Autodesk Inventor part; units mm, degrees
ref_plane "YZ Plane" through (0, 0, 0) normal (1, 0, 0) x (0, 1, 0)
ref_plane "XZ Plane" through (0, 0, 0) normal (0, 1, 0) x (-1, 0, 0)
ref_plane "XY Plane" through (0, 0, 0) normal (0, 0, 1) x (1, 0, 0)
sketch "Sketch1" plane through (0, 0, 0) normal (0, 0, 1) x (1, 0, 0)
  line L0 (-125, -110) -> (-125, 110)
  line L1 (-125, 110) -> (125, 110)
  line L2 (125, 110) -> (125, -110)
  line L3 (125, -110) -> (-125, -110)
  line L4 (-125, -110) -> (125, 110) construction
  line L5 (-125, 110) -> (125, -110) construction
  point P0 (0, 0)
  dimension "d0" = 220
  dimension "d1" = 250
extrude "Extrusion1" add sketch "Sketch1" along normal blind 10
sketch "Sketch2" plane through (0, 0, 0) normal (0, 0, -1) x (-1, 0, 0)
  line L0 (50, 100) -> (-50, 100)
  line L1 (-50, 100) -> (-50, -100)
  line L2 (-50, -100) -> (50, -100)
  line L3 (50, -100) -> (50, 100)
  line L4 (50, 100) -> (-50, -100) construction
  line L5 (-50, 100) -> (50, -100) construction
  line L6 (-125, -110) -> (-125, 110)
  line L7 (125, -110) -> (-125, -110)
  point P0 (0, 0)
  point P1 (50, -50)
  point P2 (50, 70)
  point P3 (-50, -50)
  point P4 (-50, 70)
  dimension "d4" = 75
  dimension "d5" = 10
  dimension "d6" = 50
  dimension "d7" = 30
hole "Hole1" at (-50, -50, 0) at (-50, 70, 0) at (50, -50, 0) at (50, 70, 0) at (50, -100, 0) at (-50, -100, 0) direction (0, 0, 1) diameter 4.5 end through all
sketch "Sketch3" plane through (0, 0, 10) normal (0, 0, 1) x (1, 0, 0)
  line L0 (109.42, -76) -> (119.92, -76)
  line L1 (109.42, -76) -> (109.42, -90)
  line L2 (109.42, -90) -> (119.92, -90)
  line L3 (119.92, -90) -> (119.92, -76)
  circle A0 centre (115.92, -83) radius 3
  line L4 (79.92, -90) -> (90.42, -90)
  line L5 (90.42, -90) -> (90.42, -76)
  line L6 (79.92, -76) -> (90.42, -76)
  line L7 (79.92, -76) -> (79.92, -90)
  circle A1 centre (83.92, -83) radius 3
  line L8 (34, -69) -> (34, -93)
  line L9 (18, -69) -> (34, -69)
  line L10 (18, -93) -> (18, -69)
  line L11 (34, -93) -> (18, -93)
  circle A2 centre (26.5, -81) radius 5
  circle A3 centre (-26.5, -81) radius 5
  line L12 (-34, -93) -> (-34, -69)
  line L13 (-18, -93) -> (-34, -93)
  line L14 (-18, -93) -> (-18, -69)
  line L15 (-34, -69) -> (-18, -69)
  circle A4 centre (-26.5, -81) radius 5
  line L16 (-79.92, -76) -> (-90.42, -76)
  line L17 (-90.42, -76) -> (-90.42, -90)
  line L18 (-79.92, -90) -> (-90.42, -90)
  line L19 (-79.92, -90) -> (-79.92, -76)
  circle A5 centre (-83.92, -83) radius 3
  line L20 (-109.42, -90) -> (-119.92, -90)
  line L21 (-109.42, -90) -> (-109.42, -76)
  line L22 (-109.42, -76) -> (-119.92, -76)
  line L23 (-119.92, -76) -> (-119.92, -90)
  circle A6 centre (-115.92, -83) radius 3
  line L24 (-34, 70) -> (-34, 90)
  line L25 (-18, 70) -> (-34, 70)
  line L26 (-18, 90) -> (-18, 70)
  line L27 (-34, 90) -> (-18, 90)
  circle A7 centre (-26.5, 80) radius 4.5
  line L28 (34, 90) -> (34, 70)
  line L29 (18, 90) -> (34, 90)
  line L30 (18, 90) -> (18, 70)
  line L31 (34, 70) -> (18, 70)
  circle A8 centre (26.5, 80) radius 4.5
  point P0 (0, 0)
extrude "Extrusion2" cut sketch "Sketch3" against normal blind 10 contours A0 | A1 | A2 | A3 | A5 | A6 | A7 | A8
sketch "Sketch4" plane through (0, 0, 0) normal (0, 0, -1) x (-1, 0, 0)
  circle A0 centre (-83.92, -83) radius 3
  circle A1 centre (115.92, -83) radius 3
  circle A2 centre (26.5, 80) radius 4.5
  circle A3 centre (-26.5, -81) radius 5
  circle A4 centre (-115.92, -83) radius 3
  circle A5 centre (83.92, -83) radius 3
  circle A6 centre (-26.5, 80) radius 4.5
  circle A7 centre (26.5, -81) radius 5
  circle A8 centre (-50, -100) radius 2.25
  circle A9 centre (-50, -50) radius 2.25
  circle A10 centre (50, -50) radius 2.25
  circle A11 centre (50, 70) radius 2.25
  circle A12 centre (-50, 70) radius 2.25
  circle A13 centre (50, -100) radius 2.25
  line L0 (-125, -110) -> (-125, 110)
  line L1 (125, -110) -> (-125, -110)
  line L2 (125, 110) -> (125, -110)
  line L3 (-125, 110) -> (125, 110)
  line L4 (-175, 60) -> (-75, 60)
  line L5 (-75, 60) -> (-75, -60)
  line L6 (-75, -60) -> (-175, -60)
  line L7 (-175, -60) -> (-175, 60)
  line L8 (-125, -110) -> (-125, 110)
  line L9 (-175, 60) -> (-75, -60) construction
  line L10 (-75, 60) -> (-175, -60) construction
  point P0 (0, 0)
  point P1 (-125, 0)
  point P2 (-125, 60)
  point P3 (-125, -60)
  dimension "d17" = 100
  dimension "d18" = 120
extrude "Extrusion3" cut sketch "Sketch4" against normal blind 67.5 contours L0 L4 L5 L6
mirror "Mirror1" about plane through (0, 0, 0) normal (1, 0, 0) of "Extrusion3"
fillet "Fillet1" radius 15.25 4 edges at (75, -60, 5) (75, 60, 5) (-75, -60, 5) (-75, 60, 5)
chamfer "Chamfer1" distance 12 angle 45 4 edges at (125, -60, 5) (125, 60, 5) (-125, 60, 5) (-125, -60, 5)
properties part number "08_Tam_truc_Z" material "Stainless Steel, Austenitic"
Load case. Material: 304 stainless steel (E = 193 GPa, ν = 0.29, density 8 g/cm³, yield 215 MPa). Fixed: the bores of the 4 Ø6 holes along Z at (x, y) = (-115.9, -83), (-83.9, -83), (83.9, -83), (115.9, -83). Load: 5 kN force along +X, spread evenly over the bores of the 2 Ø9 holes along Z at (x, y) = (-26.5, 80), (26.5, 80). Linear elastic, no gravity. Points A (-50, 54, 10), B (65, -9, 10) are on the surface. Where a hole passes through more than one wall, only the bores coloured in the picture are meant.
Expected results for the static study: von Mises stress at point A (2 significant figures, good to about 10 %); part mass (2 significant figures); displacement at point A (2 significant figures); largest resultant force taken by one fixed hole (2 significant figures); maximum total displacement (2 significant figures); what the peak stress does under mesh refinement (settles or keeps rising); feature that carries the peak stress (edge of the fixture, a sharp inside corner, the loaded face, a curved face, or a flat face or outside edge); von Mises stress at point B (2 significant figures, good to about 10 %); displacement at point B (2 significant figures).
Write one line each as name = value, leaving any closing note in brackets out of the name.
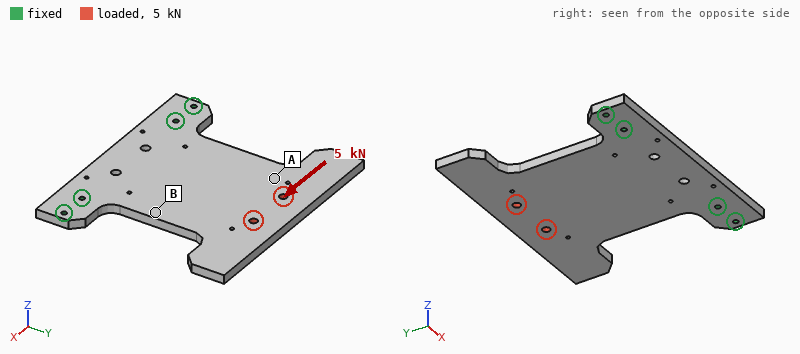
von Mises stress at point A = 5.8 MPa
part mass = 3.4 kg
displacement at point A = 19 µm
largest resultant force taken by one fixed hole = 4.9 kN
maximum total displacement = 33 µm
what the peak stress does under mesh refinement = keeps rising
feature that carries the peak stress = edge of the fixture
von Mises stress at point B = 11 MPa
displacement at point B = 10 µm
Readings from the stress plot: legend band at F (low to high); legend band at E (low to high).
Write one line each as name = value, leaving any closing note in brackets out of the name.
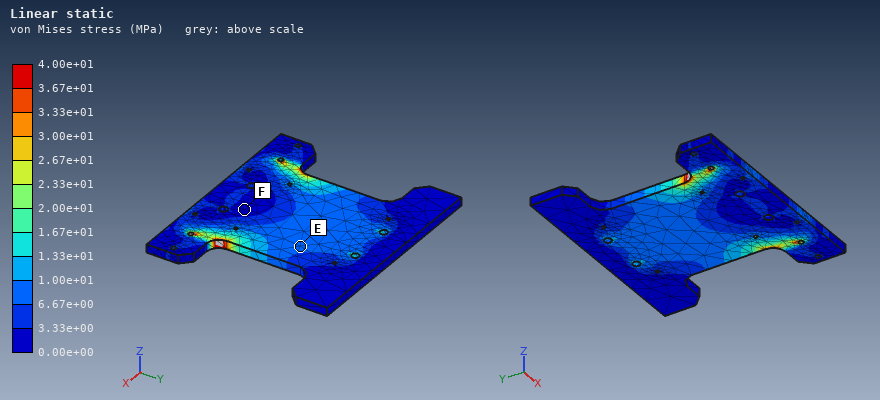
legend band at F = 0.00e+00 to 3.33e+00 MPa
legend band at E = 6.67e+00 to 1.00e+01 MPa
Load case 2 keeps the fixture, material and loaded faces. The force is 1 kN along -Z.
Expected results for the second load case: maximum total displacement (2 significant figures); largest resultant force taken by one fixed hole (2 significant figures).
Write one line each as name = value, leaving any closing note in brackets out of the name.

maximum total displacement = 1.1 mm
largest resultant force taken by one fixed hole = 700 N
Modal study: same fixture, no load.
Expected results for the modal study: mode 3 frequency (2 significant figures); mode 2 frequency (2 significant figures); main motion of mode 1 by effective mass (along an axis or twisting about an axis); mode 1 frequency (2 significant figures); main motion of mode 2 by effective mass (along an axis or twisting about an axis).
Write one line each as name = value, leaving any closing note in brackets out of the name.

mode 3 frequency = 950 Hz
mode 2 frequency = 360 Hz
main motion of mode 1 by effective mass = along Z
mode 1 frequency = 140 Hz
main motion of mode 2 by effective mass = twisting about Y
